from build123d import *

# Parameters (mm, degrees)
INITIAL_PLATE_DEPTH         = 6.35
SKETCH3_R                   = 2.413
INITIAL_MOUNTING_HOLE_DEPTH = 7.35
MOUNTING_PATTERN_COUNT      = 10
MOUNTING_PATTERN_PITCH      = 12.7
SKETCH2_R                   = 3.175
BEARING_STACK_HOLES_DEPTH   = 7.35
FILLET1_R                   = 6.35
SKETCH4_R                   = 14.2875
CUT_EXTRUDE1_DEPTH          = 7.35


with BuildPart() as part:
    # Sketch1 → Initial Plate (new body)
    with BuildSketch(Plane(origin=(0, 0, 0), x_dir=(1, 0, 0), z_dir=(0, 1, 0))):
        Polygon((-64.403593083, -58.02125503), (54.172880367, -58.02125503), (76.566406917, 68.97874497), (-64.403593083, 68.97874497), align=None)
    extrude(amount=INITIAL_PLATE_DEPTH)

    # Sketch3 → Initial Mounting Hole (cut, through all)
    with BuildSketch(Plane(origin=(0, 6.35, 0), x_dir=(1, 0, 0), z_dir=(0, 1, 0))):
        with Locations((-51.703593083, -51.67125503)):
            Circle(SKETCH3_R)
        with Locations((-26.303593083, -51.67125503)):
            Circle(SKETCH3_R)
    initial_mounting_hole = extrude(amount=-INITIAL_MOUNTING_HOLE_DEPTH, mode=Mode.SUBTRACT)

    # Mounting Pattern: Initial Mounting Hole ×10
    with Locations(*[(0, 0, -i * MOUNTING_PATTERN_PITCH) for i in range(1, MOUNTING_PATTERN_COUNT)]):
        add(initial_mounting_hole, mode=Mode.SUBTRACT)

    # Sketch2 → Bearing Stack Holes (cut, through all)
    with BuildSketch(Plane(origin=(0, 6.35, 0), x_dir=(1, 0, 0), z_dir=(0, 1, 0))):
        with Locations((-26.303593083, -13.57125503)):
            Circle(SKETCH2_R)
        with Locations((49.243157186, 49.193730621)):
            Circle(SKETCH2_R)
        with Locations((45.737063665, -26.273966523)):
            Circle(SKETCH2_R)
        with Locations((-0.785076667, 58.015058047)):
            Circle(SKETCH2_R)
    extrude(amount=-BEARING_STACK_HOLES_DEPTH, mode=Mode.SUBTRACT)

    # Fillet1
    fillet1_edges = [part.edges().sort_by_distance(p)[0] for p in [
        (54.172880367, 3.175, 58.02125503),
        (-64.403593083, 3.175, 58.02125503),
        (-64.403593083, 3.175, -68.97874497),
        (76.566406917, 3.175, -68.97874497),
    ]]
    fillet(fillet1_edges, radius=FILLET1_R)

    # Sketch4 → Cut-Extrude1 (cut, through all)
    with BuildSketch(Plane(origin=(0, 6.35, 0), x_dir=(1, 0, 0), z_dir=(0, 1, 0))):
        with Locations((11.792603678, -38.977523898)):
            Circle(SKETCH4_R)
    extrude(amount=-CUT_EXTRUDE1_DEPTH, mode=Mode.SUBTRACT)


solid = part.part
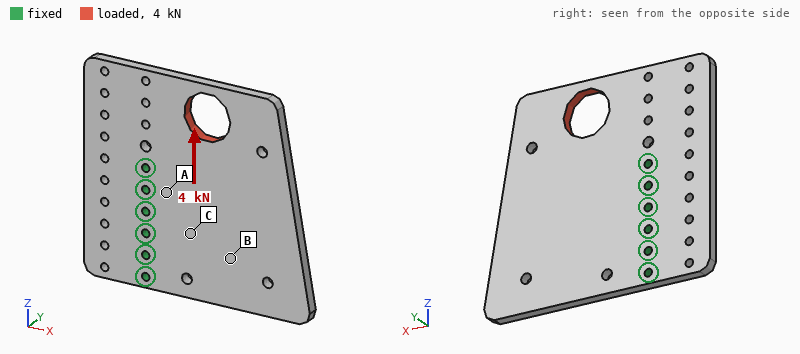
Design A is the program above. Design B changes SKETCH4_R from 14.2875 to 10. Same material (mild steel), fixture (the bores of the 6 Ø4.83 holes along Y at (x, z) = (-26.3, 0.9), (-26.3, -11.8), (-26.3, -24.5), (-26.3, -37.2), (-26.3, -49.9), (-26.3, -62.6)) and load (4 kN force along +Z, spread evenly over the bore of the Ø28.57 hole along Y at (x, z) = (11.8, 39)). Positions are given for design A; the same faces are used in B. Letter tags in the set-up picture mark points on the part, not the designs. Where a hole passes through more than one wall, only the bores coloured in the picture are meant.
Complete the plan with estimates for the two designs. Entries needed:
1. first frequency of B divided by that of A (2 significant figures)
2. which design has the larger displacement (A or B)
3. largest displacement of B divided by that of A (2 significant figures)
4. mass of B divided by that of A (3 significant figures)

1.0
A
0.84
1.02
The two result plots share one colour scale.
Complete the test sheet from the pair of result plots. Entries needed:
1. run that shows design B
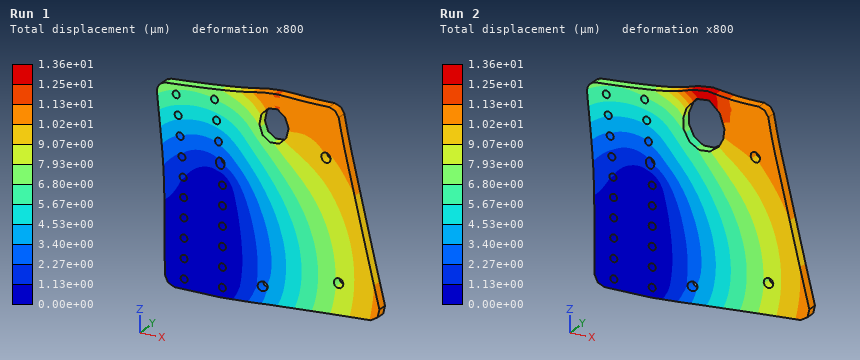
Run 1
